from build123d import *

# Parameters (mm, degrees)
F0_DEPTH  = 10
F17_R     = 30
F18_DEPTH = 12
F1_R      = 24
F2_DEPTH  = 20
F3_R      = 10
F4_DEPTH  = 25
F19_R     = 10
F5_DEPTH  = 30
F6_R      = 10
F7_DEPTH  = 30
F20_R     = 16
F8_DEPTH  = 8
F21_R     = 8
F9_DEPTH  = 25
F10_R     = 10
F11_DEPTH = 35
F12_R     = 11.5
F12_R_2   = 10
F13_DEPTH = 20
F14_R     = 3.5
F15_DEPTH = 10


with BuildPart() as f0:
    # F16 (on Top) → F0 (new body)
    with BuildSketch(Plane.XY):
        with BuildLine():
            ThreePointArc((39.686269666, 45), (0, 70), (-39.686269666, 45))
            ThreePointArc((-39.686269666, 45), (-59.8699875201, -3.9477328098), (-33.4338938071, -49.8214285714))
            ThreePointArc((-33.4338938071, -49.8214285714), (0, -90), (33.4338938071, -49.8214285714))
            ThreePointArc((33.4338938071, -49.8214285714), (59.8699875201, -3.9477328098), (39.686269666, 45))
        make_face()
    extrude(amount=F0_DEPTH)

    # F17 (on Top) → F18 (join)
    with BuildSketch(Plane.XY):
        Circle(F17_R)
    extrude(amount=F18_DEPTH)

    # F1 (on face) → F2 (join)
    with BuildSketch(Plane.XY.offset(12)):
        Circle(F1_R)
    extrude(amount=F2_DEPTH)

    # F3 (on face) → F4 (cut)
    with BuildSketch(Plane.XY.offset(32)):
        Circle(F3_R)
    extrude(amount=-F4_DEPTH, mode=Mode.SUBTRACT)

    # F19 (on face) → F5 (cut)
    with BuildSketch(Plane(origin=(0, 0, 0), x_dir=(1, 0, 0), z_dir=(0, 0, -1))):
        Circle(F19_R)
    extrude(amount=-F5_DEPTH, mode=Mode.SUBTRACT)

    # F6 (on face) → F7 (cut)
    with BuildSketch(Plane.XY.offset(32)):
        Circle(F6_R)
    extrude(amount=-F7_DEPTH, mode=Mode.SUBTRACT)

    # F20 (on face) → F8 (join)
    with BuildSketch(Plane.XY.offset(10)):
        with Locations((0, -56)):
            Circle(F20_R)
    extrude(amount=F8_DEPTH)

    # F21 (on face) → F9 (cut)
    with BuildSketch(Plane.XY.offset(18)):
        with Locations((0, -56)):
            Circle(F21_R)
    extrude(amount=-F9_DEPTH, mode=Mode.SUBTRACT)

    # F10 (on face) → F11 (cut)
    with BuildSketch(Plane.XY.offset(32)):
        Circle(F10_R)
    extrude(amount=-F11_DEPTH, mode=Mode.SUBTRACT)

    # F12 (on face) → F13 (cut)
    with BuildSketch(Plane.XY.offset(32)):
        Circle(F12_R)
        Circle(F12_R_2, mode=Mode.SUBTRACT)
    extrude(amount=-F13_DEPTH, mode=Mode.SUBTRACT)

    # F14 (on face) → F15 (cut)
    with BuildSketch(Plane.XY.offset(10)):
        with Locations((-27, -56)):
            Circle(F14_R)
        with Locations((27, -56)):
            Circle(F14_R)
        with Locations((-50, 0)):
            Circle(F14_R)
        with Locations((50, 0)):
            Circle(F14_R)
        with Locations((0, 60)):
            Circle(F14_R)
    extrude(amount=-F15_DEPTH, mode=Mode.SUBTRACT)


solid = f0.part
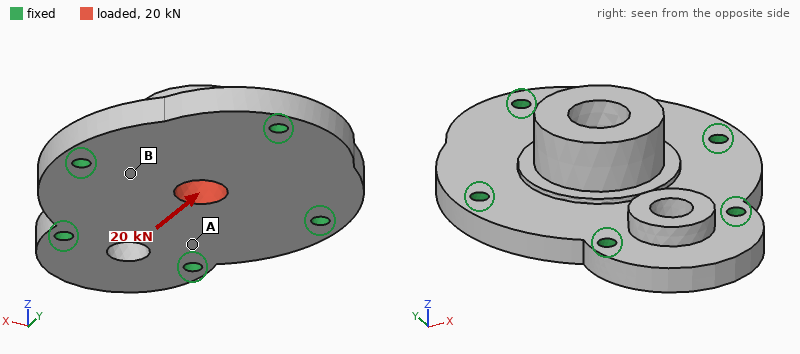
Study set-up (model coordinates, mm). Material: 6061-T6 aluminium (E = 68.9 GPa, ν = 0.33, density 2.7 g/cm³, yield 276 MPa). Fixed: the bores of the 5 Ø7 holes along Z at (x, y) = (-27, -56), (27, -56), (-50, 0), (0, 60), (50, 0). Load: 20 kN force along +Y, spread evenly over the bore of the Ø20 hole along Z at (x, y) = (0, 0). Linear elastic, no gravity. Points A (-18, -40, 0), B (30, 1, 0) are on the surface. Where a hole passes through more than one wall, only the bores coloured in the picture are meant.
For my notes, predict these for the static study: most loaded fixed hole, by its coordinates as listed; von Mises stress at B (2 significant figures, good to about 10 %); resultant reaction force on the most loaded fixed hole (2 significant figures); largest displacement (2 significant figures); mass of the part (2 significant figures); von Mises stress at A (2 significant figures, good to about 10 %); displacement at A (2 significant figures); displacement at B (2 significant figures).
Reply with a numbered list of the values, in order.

1. (0, 60)
2. 6.7 MPa
3. 5.2 kN
4. 17 µm
5. 450 g
6. 19 MPa
7. 5.4 µm
8. 6.7 µm
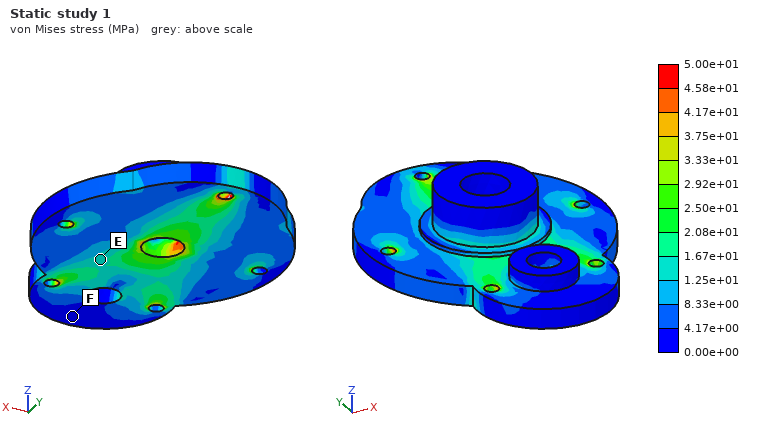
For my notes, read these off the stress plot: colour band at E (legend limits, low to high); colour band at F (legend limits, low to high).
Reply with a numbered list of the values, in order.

1. 1.25e+01 to 1.67e+01 MPa
2. 0.00e+00 to 4.17e+00 MPa
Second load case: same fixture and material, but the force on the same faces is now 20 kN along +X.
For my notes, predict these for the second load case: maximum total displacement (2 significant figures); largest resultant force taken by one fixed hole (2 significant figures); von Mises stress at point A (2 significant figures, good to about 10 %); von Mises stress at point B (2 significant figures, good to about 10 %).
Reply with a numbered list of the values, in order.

1. 17 µm
2. 6.8 kN
3. 10 MPa
4. 26 MPa
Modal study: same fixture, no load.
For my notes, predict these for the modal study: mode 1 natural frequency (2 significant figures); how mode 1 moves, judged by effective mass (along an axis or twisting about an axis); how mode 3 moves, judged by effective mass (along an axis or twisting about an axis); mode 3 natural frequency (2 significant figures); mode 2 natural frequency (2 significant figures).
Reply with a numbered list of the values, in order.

1. 5400 Hz
2. along Z
3. twisting about Y
4. 7400 Hz
5. 6900 Hz
